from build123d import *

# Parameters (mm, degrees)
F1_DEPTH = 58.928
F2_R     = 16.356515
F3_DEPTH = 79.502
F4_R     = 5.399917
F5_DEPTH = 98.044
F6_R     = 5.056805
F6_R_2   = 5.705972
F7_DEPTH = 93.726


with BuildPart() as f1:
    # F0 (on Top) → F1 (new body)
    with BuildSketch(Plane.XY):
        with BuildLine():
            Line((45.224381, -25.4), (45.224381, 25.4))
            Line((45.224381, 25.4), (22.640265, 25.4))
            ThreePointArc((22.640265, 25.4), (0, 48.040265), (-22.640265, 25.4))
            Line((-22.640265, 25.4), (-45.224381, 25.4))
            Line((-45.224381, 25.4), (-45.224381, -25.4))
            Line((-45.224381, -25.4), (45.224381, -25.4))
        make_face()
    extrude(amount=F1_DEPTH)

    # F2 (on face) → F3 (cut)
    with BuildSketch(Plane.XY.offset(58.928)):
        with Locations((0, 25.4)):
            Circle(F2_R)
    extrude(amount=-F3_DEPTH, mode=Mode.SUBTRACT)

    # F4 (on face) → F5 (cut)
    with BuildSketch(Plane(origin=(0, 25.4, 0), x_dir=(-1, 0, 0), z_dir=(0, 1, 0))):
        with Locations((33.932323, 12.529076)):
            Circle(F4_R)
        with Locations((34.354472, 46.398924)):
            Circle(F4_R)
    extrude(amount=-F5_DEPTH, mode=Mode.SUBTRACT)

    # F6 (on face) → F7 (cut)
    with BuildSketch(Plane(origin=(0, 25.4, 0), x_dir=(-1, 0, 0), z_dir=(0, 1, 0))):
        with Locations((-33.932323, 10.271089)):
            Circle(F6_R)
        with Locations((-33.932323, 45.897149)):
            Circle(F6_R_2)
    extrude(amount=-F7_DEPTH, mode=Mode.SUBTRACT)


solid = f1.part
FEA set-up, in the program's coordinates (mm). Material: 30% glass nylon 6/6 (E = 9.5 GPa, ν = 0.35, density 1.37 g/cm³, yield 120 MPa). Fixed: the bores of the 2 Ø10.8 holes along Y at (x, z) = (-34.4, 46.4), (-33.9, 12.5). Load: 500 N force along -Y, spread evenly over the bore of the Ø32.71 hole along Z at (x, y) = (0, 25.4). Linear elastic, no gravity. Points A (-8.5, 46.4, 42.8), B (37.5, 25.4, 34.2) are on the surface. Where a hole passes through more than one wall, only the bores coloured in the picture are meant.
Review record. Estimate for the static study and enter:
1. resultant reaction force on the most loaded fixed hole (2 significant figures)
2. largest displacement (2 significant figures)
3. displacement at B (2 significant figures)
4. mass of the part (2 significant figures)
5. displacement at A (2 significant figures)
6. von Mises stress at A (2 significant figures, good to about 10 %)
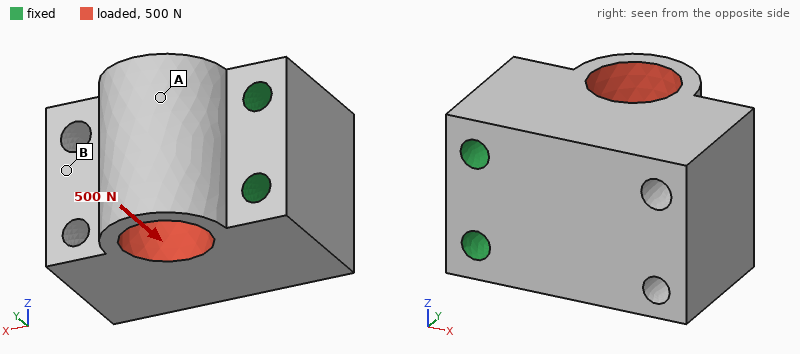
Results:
250 N
10 µm
9.3 µm
340 g
7.1 µm
0.42 MPa
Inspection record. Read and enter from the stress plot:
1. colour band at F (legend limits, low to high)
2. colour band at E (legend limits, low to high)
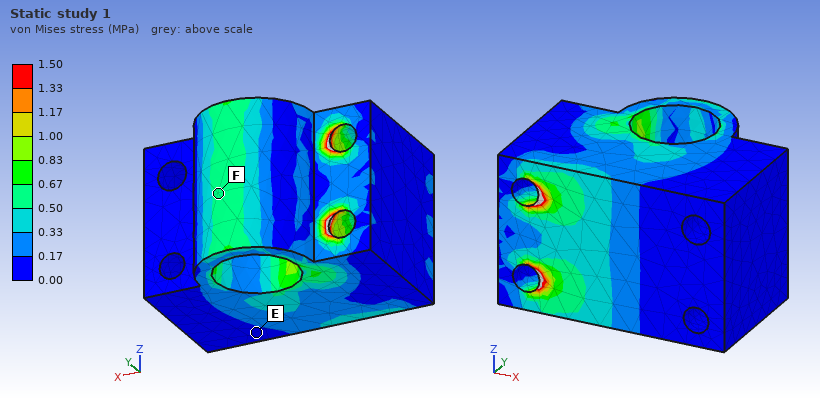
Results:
0.50 to 0.67 MPa
0.00 to 0.17 MPa
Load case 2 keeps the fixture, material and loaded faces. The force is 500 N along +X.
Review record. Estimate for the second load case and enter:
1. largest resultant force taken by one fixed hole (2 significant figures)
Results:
250 N
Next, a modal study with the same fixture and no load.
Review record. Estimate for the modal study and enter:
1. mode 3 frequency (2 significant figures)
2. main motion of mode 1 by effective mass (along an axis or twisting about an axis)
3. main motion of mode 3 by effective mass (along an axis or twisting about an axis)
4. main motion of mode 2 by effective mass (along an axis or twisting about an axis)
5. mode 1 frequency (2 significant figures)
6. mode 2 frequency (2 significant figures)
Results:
4200 Hz
along Y
twisting about X
along Z
2200 Hz
2800 Hz
